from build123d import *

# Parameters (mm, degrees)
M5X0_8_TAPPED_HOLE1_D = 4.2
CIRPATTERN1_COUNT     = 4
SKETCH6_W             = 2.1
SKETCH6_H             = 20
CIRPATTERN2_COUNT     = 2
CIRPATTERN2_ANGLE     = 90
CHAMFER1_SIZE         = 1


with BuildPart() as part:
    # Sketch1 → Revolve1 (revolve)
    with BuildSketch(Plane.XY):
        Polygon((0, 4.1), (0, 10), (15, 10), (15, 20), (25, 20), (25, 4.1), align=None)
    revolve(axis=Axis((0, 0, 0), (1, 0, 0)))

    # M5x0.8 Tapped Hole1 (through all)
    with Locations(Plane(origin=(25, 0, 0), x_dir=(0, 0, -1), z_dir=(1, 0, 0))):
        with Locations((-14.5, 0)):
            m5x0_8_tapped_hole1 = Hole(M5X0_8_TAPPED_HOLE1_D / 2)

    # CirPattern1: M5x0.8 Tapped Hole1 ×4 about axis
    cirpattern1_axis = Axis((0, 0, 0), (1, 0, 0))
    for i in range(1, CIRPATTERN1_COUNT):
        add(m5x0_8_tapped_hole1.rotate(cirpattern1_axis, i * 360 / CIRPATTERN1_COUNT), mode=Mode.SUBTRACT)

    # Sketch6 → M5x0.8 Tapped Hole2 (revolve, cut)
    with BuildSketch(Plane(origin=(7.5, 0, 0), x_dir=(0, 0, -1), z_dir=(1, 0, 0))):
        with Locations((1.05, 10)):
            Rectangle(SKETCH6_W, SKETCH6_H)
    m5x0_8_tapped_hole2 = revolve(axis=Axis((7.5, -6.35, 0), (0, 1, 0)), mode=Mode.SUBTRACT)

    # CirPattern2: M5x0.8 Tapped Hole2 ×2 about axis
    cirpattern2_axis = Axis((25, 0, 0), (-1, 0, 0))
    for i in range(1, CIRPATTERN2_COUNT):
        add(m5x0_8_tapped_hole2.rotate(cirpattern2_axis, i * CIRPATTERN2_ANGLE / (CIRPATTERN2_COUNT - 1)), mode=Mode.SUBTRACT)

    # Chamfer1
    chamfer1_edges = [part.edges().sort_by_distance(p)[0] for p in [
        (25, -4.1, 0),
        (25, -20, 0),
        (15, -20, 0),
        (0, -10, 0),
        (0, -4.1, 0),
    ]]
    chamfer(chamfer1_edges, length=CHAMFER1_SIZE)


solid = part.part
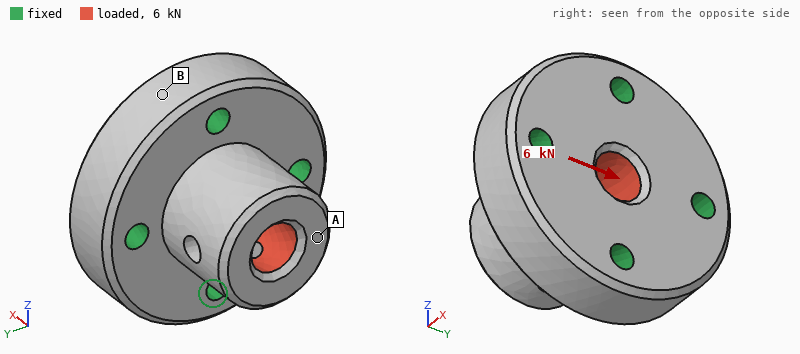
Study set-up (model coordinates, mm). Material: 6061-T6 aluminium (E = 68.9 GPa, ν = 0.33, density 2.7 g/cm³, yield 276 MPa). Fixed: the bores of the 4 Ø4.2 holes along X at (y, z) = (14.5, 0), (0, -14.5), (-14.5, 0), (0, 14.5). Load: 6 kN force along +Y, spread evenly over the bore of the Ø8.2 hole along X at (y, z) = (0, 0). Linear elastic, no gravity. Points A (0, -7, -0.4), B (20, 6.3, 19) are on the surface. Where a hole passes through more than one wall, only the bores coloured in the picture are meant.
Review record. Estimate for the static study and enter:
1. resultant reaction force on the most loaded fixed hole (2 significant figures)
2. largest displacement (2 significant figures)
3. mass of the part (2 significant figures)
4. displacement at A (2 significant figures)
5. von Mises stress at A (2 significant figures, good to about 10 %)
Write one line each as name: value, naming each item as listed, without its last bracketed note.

resultant reaction force on the most loaded fixed hole: 2.4 kN
largest displacement: 17 µm
mass of the part: 41 g
displacement at A: 17 µm
von Mises stress at A: 13 MPa
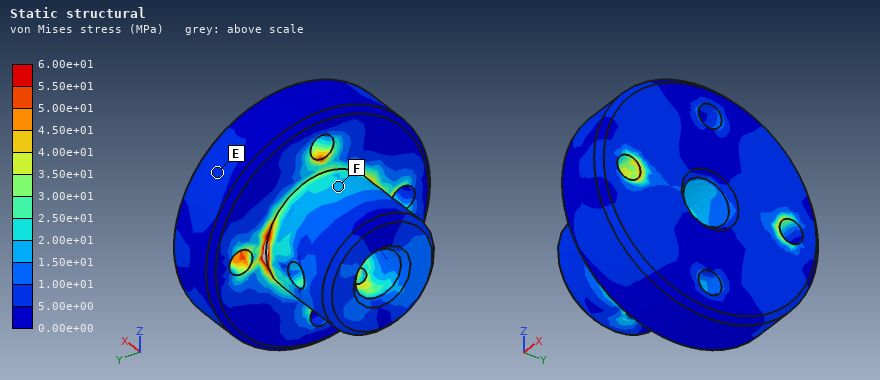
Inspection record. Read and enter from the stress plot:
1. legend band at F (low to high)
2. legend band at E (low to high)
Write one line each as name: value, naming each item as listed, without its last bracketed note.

legend band at F: 1.50e+01 to 2.00e+01 MPa
legend band at E: 5.00e+00 to 1.00e+01 MPa
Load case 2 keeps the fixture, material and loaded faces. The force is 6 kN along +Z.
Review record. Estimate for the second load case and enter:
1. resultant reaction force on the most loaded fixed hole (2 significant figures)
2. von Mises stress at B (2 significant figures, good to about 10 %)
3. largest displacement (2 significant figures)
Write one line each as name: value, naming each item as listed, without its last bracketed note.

resultant reaction force on the most loaded fixed hole: 2.4 kN
von Mises stress at B: 5.5 MPa
largest displacement: 17 µm
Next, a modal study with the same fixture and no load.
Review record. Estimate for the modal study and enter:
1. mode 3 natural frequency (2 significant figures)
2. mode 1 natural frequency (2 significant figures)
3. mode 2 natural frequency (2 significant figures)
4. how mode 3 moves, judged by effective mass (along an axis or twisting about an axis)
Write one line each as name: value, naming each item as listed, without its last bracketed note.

mode 3 natural frequency: 42 kHz
mode 1 natural frequency: 26 kHz
mode 2 natural frequency: 26 kHz
how mode 3 moves, judged by effective mass: along X
